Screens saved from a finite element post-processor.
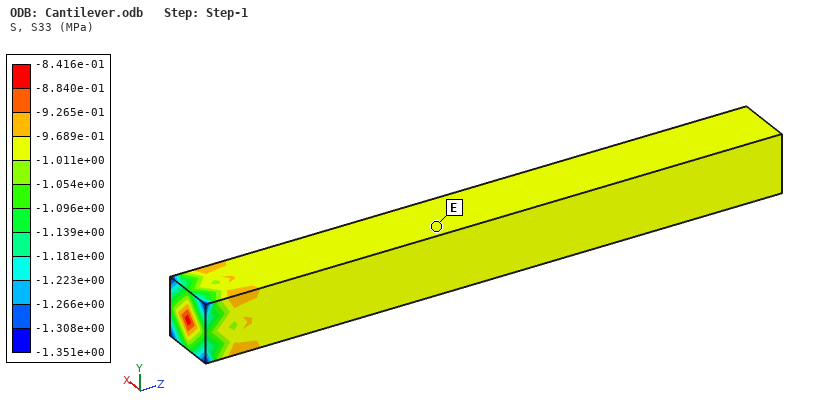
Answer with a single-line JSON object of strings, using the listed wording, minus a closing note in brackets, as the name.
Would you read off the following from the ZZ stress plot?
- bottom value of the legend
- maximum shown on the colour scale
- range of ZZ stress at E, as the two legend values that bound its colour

{"bottom value of the legend": "-1.351e+00 MPa", "maximum shown on the colour scale": "-8.416e-01 MPa", "range of ZZ stress at E, as the two legend values that bound its colour": "-1.011e+00 to -9.689e-01 MPa"}
